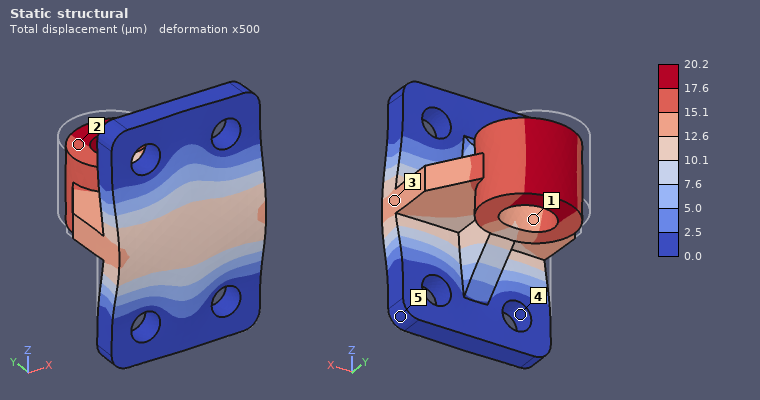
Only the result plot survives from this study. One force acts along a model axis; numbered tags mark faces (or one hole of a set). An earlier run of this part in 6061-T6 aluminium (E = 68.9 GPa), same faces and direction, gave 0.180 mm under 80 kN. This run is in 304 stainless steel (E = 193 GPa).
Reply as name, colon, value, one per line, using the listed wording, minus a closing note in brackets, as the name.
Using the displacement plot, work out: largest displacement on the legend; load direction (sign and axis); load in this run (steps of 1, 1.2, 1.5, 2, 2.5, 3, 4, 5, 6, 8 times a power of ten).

largest displacement on the legend: 20.2 µm
load direction: -Y
load in this run: 25 kN
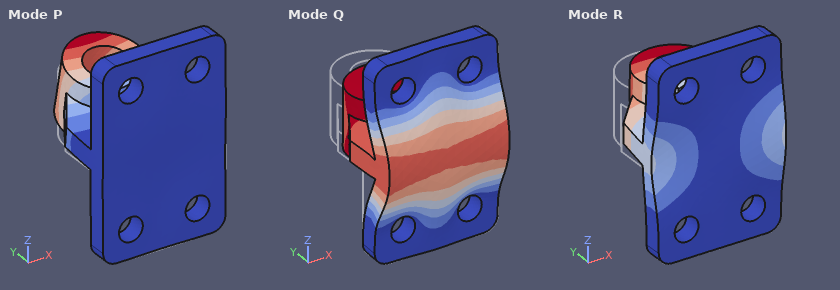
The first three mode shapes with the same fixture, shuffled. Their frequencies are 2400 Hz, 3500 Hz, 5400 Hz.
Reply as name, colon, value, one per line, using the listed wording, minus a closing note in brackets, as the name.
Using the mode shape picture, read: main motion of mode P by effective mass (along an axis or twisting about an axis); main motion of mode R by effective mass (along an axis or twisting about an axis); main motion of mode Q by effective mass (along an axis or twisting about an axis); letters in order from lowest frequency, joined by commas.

main motion of mode P by effective mass: along Z
main motion of mode R by effective mass: along X
main motion of mode Q by effective mass: along Y
letters in order from lowest frequency, joined by commas: R, P, Q
